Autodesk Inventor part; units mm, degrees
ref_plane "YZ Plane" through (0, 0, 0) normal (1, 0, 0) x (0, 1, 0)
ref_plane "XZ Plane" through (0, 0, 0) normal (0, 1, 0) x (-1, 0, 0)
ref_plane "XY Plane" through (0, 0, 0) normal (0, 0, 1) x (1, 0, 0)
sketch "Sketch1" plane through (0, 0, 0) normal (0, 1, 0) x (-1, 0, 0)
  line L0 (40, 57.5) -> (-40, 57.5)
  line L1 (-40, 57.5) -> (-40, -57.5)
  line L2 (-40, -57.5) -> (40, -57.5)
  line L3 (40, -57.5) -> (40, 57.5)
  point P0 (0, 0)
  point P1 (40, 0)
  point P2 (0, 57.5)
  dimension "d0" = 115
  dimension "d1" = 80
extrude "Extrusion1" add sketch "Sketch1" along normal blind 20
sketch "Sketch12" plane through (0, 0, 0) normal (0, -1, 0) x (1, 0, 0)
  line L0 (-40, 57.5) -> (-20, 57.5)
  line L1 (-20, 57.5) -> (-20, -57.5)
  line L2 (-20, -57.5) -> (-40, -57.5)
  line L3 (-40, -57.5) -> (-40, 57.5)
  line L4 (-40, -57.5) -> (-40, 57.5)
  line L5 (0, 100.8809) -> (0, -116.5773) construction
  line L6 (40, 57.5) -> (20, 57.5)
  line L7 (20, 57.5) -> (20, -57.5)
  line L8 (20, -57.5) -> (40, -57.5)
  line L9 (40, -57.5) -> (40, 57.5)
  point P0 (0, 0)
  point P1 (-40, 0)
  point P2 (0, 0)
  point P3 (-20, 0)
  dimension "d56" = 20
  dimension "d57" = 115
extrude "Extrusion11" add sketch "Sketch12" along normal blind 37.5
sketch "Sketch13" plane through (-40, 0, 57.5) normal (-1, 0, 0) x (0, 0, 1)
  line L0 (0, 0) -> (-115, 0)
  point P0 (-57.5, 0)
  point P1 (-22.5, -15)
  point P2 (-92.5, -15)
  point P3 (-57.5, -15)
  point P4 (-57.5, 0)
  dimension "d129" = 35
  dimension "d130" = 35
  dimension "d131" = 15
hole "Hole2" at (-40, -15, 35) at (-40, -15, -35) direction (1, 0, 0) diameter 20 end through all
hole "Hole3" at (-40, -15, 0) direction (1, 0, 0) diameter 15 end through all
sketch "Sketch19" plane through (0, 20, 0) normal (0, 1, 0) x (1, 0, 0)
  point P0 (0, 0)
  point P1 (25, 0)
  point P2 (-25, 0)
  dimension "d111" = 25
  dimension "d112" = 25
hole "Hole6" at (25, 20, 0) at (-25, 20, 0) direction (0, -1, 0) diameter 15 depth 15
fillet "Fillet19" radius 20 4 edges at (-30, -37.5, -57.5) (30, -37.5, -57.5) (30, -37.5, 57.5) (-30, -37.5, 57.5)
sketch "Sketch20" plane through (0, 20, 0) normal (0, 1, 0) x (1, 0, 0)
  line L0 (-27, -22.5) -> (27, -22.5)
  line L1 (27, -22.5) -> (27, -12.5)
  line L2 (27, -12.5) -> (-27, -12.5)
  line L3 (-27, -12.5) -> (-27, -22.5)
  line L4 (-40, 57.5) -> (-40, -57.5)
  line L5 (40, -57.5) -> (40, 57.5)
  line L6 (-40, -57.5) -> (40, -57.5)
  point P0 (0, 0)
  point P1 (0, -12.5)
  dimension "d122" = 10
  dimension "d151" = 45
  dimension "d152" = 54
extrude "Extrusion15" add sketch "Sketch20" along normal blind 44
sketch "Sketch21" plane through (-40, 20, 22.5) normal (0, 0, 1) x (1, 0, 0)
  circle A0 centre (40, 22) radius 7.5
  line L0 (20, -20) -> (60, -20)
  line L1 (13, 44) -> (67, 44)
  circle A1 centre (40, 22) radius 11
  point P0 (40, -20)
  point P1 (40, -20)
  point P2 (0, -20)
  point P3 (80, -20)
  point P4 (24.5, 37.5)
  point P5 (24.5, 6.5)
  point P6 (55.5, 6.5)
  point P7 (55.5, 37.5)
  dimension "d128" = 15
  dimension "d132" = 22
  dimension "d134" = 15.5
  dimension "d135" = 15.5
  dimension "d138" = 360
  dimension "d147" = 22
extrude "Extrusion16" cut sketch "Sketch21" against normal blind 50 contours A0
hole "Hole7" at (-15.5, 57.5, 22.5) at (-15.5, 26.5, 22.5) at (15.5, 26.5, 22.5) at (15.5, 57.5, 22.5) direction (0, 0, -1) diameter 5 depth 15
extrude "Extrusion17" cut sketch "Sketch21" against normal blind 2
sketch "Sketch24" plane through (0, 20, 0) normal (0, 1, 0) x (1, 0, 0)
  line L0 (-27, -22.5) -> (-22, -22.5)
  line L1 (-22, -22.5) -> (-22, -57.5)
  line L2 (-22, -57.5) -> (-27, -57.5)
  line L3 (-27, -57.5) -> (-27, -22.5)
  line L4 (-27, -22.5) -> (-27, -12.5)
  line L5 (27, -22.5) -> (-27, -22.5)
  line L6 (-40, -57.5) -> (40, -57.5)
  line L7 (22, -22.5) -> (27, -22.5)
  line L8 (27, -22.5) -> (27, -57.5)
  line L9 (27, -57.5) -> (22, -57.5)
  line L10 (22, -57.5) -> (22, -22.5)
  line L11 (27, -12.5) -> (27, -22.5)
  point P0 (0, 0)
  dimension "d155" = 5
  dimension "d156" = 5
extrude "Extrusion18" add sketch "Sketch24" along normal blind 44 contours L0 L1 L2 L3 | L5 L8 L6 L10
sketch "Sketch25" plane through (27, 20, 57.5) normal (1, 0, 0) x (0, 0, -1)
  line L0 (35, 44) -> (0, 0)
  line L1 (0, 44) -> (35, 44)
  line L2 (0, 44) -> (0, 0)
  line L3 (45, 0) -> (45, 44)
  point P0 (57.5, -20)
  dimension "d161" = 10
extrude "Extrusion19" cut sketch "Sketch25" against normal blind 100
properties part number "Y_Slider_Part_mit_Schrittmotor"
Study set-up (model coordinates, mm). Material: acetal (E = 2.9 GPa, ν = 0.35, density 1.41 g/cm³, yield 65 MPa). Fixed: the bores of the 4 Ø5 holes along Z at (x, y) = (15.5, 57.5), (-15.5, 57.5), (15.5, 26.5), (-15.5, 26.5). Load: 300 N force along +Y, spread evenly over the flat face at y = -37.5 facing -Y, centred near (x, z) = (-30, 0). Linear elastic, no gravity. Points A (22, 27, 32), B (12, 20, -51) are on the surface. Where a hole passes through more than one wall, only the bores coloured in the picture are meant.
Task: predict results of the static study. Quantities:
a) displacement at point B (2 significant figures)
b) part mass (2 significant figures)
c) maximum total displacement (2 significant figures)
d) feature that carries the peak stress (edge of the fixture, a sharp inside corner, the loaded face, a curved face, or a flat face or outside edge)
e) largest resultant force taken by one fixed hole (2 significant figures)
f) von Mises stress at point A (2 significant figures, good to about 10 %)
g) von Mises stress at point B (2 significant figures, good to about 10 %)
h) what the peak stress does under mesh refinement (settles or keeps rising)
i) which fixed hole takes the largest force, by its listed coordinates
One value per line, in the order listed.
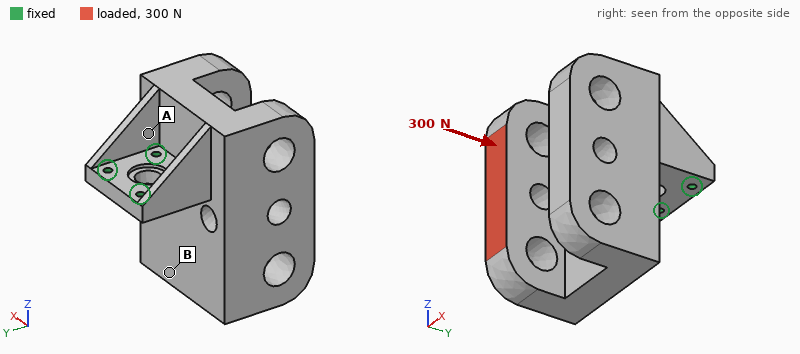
0.097 mm
480 g
0.18 mm
edge of the fixture
360 N
0.86 MPa
0.26 MPa
keeps rising
(-15.5, 26.5)
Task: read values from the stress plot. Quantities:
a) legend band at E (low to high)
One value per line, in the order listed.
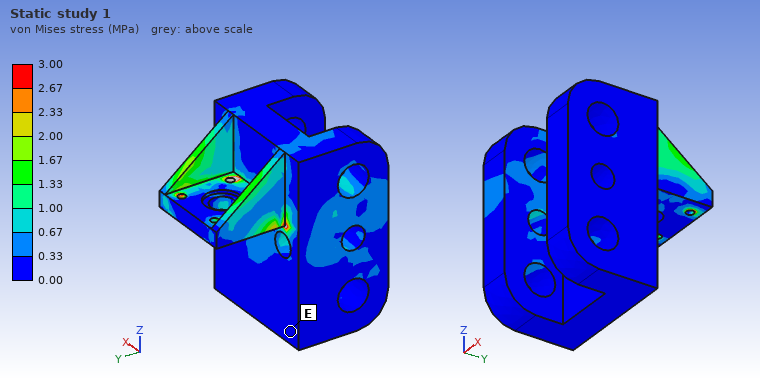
0.00 to 0.33 MPa
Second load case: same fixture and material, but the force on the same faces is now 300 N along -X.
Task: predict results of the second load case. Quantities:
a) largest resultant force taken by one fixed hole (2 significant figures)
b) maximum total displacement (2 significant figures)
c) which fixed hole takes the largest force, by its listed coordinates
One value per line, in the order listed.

520 N
0.24 mm
(15.5, 26.5)
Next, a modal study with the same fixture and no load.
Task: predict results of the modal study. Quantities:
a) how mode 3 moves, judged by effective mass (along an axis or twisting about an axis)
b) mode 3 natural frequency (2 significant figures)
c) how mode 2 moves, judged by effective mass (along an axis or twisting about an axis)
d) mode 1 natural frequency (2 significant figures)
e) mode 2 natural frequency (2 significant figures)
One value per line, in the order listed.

along X
710 Hz
along X
310 Hz
490 Hz
